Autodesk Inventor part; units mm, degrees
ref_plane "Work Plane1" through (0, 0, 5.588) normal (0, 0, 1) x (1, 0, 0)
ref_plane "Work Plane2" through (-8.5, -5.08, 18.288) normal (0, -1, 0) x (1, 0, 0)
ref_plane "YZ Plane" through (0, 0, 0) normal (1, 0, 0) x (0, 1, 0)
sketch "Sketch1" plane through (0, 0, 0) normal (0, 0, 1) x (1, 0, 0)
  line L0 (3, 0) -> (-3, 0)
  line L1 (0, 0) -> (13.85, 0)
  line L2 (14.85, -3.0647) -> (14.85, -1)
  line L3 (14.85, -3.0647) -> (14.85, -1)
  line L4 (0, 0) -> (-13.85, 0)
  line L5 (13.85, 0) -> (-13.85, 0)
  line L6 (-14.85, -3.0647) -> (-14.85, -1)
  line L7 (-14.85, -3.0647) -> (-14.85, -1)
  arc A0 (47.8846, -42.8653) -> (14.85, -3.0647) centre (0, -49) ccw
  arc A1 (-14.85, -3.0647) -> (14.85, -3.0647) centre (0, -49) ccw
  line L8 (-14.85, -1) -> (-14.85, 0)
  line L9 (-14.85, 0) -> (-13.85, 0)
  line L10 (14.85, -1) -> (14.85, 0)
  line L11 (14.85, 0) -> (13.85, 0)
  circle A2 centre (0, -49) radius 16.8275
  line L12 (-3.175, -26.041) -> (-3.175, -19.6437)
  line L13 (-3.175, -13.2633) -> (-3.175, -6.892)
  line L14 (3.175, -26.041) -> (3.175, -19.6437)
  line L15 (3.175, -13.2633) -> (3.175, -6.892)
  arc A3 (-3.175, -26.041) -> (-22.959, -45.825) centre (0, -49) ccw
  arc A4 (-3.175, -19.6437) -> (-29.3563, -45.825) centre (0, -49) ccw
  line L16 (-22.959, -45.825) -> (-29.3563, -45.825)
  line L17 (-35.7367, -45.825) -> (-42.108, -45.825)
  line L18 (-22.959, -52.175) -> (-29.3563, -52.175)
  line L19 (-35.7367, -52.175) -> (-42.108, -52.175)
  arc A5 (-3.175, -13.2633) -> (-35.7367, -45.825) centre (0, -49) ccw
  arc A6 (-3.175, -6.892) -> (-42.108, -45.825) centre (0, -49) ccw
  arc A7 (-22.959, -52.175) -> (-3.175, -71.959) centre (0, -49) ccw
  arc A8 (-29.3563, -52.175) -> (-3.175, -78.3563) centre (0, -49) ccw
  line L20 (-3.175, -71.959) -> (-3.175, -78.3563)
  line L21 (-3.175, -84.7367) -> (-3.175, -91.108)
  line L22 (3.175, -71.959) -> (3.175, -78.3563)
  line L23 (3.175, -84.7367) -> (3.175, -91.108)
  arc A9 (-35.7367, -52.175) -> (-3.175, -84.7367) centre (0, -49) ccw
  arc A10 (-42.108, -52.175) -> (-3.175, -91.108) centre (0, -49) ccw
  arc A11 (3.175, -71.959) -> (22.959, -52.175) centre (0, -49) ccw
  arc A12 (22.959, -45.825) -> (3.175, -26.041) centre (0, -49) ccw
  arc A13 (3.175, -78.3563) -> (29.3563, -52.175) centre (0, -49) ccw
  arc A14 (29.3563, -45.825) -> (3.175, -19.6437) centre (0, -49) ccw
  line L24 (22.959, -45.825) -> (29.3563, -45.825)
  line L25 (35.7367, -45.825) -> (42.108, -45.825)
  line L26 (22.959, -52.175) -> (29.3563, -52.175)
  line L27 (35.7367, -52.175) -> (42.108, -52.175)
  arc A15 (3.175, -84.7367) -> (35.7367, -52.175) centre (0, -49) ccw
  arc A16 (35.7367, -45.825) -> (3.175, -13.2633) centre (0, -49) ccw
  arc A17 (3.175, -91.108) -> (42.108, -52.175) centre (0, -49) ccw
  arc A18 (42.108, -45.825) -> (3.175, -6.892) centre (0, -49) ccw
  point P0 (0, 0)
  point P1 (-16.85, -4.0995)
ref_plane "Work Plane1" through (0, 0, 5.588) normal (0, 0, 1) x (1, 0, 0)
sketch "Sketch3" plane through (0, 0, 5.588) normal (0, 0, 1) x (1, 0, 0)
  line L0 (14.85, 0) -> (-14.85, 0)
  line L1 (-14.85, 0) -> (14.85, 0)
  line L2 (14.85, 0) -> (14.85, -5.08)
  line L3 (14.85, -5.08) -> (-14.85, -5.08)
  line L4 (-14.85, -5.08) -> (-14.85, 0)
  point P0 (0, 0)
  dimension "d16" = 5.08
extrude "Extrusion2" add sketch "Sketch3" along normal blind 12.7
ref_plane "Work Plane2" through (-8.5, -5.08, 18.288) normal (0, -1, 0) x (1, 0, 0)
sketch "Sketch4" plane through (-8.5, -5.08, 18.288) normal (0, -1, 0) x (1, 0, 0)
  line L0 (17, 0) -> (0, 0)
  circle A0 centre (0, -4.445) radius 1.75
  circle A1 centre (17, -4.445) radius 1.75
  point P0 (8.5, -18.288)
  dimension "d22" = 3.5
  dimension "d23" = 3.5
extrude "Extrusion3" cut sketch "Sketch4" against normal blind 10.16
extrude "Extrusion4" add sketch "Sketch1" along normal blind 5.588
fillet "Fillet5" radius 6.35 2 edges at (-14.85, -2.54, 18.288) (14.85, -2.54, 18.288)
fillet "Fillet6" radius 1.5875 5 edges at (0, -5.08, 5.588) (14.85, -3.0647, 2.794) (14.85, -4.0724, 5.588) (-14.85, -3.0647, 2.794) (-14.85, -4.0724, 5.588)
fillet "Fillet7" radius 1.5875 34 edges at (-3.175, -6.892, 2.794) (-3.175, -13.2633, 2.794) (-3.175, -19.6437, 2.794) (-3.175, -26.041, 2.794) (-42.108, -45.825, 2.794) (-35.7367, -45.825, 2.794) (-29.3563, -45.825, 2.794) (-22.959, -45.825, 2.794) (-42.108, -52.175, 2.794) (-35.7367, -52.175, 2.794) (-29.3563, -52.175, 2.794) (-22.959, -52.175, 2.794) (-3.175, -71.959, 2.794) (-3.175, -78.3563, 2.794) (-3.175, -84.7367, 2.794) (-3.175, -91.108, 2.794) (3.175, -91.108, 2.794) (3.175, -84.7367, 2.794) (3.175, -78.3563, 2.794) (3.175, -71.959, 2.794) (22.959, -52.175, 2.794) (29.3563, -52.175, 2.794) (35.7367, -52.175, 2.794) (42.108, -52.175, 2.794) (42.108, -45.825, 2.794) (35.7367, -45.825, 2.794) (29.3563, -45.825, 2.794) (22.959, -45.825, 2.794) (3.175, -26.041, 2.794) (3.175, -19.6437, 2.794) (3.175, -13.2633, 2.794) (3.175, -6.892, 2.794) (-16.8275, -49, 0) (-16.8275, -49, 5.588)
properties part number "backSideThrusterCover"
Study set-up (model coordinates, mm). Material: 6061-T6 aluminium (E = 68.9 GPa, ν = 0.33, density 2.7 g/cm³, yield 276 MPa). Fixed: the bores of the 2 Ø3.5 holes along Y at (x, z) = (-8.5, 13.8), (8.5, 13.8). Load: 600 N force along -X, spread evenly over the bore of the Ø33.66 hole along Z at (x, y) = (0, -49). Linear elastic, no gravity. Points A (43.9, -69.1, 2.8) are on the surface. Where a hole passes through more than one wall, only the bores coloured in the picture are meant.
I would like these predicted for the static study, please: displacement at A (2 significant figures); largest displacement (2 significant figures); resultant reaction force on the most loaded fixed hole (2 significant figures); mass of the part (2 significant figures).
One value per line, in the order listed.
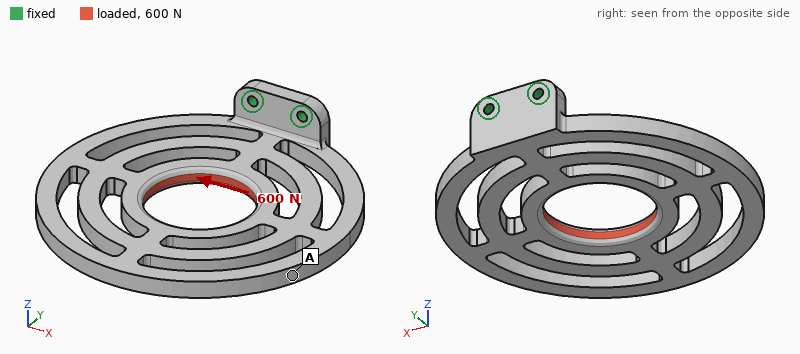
0.58 mm
0.70 mm
1.4 kN
68 g
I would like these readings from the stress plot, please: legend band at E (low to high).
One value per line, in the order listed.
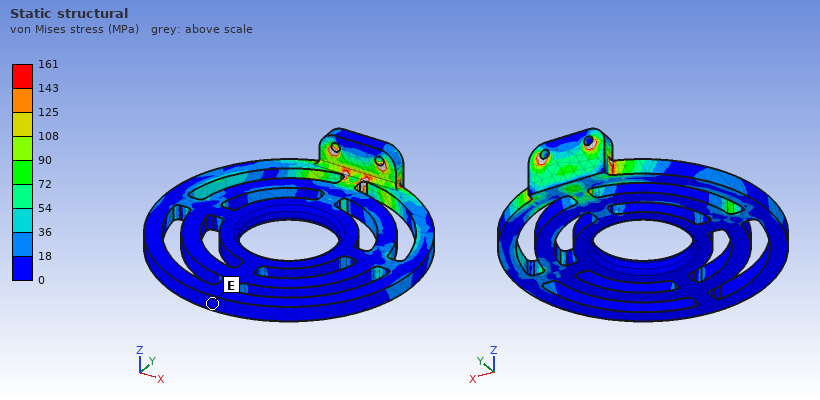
0 to 18 MPa
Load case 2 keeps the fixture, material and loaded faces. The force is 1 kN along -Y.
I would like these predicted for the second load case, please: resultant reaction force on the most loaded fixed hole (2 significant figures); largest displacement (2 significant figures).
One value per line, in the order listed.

500 N
0.29 mm
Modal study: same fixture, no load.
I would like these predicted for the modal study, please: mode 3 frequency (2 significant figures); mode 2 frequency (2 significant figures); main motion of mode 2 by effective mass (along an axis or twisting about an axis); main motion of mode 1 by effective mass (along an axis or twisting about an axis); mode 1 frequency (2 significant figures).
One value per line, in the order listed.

800 Hz
650 Hz
along X
along Z
290 Hz
